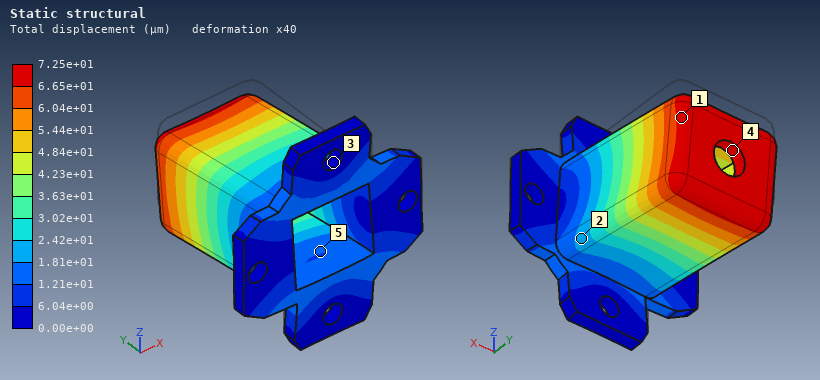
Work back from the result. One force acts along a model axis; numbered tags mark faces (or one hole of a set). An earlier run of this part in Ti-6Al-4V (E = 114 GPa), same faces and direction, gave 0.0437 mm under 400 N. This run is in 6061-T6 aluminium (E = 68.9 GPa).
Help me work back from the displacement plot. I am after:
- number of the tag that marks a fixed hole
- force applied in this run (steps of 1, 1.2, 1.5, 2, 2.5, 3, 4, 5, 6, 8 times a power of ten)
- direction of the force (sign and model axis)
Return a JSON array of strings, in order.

["3", "400 N", "-Z"]
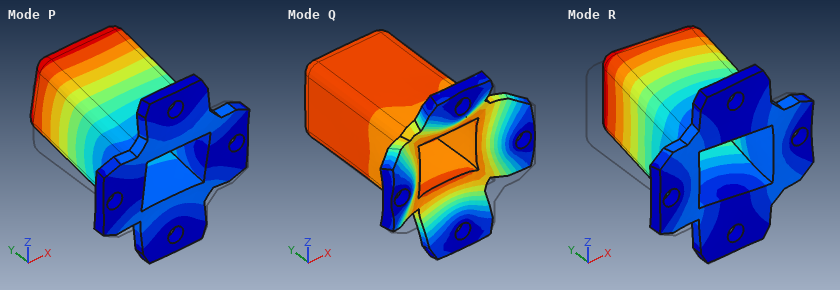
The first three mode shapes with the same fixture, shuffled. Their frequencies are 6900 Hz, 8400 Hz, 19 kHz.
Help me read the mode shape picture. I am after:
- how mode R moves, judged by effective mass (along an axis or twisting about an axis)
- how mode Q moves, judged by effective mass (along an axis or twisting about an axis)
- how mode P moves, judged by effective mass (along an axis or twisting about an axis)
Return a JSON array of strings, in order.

["along X", "along Y", "along Z"]
